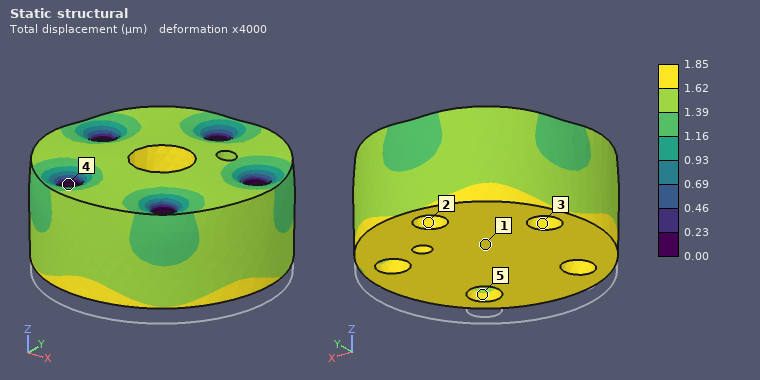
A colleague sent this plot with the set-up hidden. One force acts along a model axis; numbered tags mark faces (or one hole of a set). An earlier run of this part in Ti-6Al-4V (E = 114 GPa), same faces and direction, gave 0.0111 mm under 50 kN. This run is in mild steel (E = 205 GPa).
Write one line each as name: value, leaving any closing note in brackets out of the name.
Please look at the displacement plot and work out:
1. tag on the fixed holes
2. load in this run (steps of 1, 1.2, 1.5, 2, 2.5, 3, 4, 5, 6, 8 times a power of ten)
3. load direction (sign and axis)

tag on the fixed holes: 4
load in this run: 15 kN
load direction: +Z
